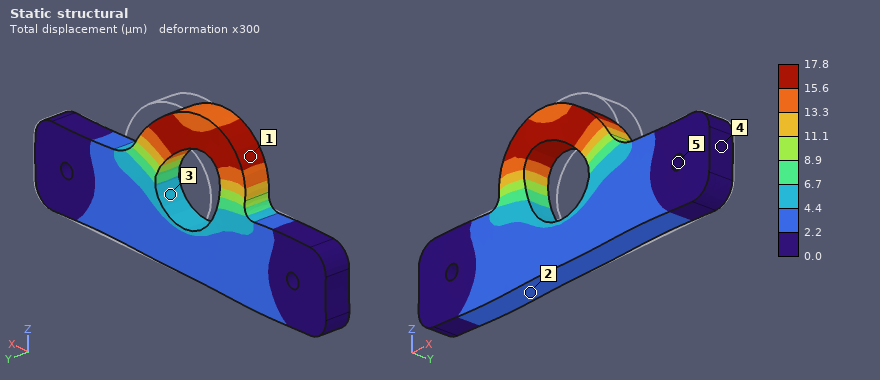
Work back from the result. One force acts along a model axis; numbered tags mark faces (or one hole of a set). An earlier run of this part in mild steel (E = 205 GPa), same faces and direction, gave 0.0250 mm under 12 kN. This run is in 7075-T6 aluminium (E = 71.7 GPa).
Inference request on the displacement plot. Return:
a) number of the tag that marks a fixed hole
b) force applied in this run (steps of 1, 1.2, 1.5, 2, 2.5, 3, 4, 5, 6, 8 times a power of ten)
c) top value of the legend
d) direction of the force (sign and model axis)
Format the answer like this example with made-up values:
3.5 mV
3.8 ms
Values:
5
3 kN
17.8 µm
-X
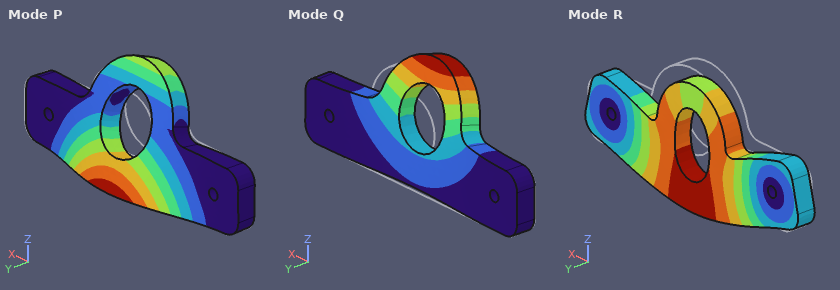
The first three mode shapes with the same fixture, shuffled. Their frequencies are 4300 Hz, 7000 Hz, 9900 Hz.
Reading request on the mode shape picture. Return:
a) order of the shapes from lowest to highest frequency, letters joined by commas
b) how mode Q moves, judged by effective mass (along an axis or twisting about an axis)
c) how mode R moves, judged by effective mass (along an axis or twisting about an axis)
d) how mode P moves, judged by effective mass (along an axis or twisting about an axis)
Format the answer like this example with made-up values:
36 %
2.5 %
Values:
Q, P, R
along Y
along Z
along Y
